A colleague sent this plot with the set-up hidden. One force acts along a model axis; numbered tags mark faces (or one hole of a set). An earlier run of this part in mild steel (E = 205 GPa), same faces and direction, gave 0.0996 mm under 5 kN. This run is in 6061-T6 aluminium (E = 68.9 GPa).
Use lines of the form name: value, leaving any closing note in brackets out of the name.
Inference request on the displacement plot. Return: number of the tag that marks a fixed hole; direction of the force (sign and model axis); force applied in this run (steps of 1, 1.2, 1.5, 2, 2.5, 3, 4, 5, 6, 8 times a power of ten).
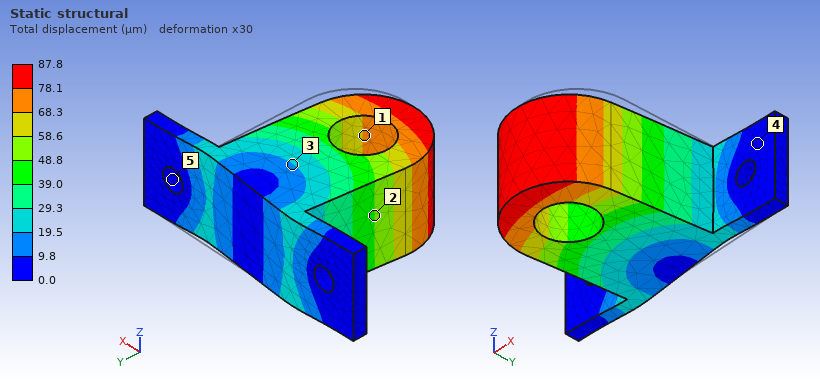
number of the tag that marks a fixed hole: 5
direction of the force: -X
force applied in this run: 1.5 kN
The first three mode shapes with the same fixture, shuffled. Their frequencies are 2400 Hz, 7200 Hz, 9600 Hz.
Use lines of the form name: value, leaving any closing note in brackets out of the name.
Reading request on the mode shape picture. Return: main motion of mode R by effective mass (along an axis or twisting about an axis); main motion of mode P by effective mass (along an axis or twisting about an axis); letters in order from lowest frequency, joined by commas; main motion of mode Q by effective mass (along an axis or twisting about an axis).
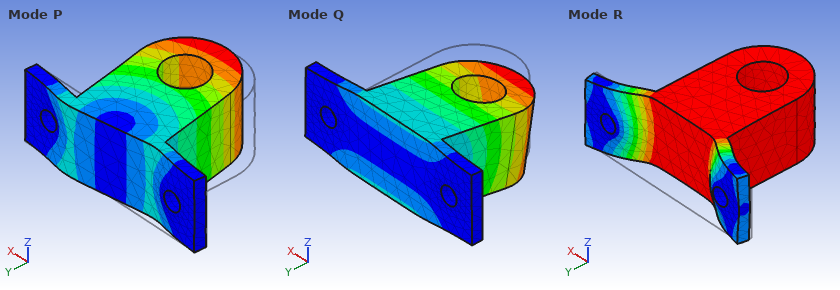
main motion of mode R by effective mass: along Y
main motion of mode P by effective mass: along X
letters in order from lowest frequency, joined by commas: Q, P, R
main motion of mode Q by effective mass: along Z
